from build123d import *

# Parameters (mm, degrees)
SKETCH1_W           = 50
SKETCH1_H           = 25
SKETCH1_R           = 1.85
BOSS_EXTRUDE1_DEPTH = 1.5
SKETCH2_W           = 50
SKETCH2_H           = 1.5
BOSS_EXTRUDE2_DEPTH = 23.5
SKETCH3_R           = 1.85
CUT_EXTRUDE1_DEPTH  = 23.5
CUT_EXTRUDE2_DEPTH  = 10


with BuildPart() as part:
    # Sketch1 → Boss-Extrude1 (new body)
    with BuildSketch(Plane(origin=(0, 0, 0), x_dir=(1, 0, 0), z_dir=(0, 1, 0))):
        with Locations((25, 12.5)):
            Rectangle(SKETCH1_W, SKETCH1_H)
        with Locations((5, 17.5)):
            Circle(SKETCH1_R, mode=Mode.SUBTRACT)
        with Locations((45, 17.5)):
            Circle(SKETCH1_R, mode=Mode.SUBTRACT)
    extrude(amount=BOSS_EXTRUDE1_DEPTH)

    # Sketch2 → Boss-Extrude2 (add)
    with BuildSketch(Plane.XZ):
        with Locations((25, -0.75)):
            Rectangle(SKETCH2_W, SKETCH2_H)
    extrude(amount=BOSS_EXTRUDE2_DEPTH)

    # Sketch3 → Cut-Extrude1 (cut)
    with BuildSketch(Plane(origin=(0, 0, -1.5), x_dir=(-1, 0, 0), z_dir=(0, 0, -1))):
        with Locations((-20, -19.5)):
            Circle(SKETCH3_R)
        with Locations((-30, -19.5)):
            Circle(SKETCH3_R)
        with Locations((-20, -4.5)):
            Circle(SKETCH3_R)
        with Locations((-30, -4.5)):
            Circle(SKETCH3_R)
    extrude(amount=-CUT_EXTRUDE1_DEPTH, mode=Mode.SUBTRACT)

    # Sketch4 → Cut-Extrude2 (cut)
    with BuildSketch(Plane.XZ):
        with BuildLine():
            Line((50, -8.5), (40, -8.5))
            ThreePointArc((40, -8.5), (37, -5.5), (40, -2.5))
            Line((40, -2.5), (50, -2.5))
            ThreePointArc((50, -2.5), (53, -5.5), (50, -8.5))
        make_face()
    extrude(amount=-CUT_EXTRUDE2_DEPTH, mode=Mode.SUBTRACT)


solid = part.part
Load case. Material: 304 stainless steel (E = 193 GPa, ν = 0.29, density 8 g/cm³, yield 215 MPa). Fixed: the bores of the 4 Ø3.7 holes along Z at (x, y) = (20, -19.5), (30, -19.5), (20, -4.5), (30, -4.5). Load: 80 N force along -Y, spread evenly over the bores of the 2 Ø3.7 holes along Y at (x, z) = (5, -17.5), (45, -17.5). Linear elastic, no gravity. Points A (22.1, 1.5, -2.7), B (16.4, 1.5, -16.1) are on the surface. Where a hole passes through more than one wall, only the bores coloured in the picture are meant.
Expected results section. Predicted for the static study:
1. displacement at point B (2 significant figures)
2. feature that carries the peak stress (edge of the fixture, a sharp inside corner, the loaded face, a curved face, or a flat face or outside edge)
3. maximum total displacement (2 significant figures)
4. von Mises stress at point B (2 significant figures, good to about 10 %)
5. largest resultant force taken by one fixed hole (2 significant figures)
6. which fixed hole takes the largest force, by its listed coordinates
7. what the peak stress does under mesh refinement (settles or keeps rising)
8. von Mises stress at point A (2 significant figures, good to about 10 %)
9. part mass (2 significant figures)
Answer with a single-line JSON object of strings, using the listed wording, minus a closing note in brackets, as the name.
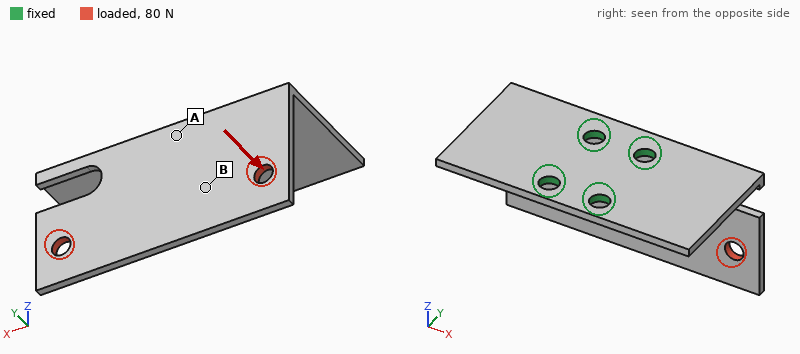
{"displacement at point B": "0.082 mm", "feature that carries the peak stress": "edge of the fixture", "maximum total displacement": "0.27 mm", "von Mises stress at point B": "22 MPa", "largest resultant force taken by one fixed hole": "36 N", "which fixed hole takes the largest force, by its listed coordinates": "(30, -4.5)", "what the peak stress does under mesh refinement": "keeps rising", "von Mises stress at point A": "67 MPa", "part mass": "27 g"}
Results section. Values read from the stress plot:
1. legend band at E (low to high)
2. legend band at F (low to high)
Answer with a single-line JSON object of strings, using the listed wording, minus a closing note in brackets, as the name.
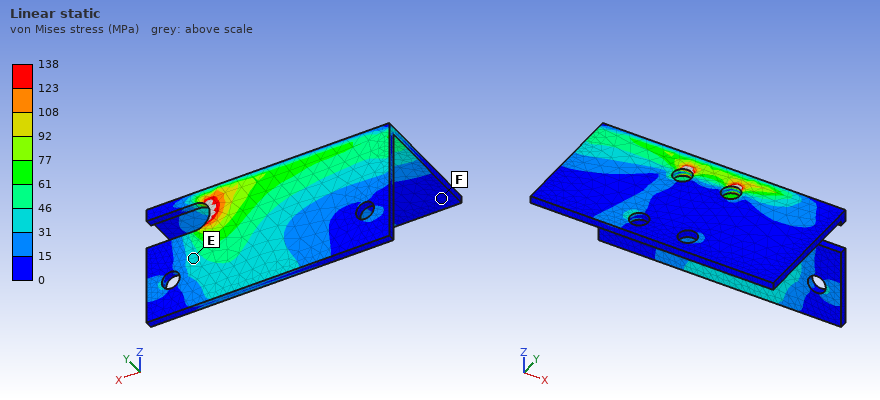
{"legend band at E": "31 to 46 MPa", "legend band at F": "0 to 15 MPa"}
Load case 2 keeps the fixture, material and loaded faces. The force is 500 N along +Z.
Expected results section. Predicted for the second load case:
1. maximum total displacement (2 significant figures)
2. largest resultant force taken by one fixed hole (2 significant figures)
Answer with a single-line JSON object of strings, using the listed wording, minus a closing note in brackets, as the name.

{"maximum total displacement": "67 µm", "largest resultant force taken by one fixed hole": "270 N"}
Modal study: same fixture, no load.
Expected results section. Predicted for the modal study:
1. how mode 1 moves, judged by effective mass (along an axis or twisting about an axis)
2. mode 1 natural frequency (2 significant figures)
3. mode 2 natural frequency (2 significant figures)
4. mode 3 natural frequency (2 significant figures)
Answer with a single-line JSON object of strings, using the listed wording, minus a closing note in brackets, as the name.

{"how mode 1 moves, judged by effective mass": "along Y", "mode 1 natural frequency": "1300 Hz", "mode 2 natural frequency": "2100 Hz", "mode 3 natural frequency": "3500 Hz"}
